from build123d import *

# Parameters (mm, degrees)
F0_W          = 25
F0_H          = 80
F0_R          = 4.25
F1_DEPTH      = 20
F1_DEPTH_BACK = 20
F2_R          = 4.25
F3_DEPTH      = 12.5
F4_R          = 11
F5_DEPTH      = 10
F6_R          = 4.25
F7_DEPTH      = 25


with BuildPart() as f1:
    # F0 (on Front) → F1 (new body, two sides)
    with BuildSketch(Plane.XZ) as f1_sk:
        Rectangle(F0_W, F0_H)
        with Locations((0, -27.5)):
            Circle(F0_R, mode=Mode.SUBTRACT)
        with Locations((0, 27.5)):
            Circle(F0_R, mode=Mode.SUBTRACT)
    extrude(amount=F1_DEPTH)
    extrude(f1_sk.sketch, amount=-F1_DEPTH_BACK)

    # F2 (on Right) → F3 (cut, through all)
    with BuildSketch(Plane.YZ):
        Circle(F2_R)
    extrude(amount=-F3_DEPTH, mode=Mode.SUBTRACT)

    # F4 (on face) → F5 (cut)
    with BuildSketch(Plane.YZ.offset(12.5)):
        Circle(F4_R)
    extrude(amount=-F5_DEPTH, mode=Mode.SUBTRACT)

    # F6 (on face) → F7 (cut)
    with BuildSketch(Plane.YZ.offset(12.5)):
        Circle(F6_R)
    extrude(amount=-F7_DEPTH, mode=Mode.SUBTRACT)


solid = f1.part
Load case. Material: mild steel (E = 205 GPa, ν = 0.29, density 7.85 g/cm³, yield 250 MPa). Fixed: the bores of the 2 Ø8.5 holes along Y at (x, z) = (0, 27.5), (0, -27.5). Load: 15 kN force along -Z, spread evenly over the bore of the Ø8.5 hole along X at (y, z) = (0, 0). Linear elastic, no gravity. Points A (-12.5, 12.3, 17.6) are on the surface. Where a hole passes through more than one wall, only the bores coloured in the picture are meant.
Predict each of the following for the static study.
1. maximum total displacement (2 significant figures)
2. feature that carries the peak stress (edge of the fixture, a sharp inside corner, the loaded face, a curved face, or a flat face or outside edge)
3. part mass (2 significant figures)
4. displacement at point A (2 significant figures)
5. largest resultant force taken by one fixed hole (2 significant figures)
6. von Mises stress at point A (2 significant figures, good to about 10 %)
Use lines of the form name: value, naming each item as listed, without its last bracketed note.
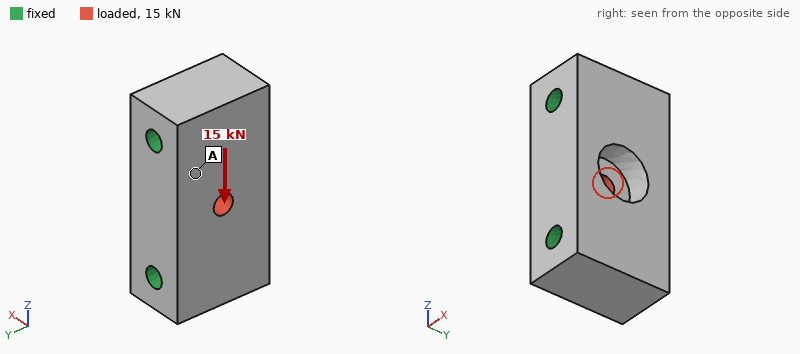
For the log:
maximum total displacement: 2.5 µm
feature that carries the peak stress: the loaded face
part mass: 560 g
displacement at point A: 0.68 µm
largest resultant force taken by one fixed hole: 7.6 kN
von Mises stress at point A: 9.0 MPa
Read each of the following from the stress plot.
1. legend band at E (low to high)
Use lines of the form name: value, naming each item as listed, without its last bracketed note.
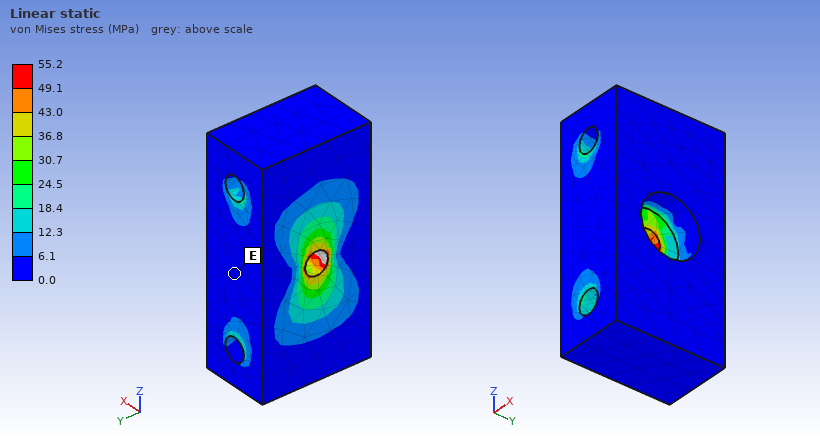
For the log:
legend band at E: 0.0 to 6.1 MPa
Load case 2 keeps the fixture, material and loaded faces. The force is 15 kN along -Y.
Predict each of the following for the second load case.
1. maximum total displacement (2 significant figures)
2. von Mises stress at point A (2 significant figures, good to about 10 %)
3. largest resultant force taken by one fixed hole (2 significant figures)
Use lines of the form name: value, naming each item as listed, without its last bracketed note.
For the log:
maximum total displacement: 5.0 µm
von Mises stress at point A: 19 MPa
largest resultant force taken by one fixed hole: 7.5 kN
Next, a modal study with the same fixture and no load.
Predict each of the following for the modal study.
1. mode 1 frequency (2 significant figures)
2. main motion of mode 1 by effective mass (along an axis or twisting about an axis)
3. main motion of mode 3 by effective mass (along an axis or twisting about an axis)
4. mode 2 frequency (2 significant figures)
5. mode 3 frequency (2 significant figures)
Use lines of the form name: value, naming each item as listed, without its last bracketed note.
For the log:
mode 1 frequency: 21 kHz
main motion of mode 1 by effective mass: along X
main motion of mode 3 by effective mass: along Y
mode 2 frequency: 27 kHz
mode 3 frequency: 28 kHz
